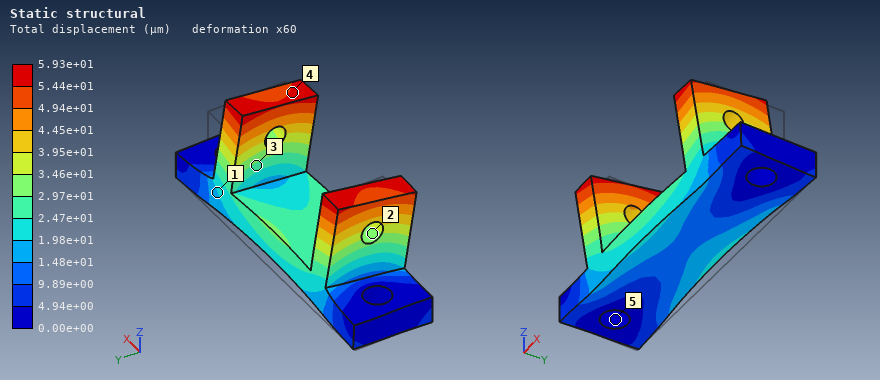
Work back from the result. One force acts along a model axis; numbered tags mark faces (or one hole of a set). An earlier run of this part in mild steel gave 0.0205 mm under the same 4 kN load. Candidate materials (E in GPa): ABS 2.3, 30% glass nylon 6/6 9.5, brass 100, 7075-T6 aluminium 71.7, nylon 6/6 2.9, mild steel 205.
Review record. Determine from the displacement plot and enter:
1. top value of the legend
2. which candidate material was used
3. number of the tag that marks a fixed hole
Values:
5.93e+01 µm
7075-T6 aluminium
5
